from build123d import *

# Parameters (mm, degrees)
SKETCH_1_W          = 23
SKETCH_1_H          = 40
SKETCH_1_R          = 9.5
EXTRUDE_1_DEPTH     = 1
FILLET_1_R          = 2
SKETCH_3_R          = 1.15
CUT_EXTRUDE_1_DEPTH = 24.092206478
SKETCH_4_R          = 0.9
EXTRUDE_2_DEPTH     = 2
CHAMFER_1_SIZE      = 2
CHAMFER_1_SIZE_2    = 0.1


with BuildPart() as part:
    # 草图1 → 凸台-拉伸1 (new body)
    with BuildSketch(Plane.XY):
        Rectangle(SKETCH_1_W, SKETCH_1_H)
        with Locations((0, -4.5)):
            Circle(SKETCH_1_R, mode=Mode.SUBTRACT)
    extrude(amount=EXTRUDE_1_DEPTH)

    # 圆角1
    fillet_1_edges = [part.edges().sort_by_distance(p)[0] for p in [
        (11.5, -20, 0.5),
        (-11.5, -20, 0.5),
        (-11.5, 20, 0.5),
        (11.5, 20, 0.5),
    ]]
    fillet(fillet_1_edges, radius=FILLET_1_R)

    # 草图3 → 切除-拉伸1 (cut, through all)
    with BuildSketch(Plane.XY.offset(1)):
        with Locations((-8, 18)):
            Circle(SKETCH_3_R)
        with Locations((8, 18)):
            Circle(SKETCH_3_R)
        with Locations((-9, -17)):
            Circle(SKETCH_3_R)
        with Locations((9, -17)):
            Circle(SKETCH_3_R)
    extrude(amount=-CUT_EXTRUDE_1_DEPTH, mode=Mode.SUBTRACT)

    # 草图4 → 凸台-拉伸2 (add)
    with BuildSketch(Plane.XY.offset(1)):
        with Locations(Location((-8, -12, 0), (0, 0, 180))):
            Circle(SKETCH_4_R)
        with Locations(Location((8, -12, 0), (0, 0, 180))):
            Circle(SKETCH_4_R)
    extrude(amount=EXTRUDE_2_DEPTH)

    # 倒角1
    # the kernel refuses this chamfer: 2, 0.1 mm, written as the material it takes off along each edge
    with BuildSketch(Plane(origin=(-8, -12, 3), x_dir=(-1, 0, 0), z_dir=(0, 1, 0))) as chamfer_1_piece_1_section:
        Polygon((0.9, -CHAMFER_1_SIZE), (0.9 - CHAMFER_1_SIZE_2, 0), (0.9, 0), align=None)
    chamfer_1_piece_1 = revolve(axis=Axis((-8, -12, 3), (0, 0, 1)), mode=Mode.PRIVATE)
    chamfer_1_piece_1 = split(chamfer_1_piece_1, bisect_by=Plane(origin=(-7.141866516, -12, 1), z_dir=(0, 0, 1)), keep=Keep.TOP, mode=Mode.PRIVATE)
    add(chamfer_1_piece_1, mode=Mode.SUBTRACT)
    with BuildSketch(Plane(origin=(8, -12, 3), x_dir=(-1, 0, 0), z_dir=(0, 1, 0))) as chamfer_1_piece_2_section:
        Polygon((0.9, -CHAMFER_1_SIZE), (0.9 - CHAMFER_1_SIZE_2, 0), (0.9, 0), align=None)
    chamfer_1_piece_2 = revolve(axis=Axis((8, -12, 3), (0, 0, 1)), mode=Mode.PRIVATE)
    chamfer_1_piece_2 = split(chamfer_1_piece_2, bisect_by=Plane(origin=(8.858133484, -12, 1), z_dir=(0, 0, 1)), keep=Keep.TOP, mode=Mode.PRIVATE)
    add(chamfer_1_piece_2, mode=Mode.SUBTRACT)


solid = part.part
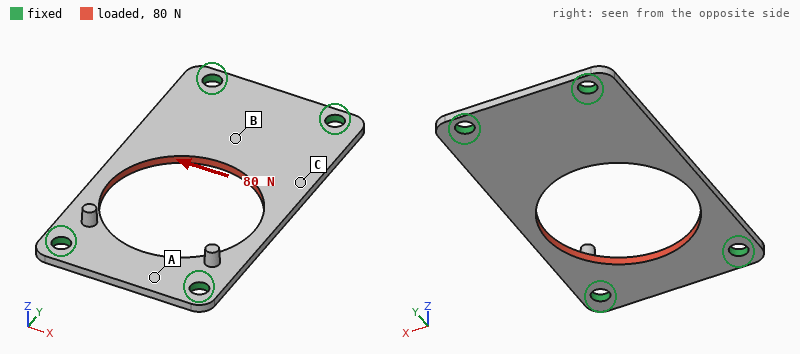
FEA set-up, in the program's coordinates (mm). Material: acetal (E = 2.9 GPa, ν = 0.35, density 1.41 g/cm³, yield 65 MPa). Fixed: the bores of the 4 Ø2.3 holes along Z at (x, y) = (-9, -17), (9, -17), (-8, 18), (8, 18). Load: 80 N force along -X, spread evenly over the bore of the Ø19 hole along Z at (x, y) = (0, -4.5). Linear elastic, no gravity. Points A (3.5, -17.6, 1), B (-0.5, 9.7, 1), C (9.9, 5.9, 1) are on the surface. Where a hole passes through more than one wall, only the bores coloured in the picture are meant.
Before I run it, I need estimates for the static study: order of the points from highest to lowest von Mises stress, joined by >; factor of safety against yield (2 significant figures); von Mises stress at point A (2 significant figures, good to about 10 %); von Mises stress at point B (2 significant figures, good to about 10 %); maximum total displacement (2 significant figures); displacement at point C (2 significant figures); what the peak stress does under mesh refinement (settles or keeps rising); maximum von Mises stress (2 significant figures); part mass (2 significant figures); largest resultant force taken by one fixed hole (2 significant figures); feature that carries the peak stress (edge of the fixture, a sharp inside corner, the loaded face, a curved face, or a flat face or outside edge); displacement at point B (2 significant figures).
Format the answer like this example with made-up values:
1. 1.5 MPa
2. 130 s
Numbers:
1. B > A > C
2. 4.7
3. 2.8 MPa
4. 5.4 MPa
5. 76 µm
6. 34 µm
7. settles
8. 14 MPa
9. 0.88 g
10. 29 N
11. a flat face or outside edge
12. 21 µm
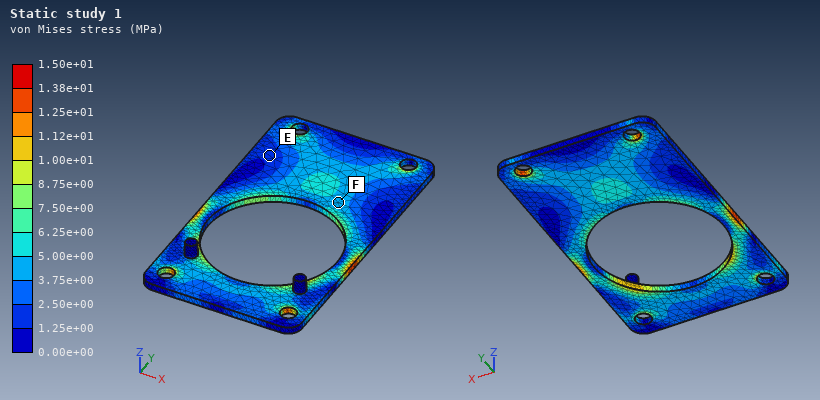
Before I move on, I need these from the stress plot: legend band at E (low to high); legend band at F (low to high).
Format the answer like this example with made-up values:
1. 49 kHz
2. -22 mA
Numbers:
1. 1.25e+00 to 2.50e+00 MPa
2. 3.75e+00 to 5.00e+00 MPa
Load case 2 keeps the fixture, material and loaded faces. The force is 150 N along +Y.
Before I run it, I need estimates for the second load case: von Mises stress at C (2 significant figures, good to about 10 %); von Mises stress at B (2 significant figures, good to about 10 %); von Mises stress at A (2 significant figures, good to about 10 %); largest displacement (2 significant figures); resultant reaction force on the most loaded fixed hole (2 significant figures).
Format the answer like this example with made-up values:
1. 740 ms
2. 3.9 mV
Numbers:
1. 3.2 MPa
2. 1.9 MPa
3. 3.3 MPa
4. 31 µm
5. 43 N
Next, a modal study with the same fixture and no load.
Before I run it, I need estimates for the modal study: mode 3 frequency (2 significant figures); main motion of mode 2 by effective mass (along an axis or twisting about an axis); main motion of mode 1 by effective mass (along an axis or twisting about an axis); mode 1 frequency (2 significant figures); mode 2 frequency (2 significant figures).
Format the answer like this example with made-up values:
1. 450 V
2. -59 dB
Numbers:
1. 3100 Hz
2. twisting about Y
3. along Z
4. 1400 Hz
5. 1800 Hz
